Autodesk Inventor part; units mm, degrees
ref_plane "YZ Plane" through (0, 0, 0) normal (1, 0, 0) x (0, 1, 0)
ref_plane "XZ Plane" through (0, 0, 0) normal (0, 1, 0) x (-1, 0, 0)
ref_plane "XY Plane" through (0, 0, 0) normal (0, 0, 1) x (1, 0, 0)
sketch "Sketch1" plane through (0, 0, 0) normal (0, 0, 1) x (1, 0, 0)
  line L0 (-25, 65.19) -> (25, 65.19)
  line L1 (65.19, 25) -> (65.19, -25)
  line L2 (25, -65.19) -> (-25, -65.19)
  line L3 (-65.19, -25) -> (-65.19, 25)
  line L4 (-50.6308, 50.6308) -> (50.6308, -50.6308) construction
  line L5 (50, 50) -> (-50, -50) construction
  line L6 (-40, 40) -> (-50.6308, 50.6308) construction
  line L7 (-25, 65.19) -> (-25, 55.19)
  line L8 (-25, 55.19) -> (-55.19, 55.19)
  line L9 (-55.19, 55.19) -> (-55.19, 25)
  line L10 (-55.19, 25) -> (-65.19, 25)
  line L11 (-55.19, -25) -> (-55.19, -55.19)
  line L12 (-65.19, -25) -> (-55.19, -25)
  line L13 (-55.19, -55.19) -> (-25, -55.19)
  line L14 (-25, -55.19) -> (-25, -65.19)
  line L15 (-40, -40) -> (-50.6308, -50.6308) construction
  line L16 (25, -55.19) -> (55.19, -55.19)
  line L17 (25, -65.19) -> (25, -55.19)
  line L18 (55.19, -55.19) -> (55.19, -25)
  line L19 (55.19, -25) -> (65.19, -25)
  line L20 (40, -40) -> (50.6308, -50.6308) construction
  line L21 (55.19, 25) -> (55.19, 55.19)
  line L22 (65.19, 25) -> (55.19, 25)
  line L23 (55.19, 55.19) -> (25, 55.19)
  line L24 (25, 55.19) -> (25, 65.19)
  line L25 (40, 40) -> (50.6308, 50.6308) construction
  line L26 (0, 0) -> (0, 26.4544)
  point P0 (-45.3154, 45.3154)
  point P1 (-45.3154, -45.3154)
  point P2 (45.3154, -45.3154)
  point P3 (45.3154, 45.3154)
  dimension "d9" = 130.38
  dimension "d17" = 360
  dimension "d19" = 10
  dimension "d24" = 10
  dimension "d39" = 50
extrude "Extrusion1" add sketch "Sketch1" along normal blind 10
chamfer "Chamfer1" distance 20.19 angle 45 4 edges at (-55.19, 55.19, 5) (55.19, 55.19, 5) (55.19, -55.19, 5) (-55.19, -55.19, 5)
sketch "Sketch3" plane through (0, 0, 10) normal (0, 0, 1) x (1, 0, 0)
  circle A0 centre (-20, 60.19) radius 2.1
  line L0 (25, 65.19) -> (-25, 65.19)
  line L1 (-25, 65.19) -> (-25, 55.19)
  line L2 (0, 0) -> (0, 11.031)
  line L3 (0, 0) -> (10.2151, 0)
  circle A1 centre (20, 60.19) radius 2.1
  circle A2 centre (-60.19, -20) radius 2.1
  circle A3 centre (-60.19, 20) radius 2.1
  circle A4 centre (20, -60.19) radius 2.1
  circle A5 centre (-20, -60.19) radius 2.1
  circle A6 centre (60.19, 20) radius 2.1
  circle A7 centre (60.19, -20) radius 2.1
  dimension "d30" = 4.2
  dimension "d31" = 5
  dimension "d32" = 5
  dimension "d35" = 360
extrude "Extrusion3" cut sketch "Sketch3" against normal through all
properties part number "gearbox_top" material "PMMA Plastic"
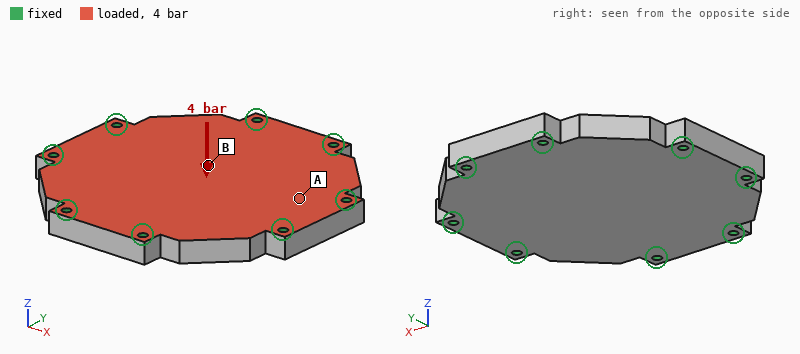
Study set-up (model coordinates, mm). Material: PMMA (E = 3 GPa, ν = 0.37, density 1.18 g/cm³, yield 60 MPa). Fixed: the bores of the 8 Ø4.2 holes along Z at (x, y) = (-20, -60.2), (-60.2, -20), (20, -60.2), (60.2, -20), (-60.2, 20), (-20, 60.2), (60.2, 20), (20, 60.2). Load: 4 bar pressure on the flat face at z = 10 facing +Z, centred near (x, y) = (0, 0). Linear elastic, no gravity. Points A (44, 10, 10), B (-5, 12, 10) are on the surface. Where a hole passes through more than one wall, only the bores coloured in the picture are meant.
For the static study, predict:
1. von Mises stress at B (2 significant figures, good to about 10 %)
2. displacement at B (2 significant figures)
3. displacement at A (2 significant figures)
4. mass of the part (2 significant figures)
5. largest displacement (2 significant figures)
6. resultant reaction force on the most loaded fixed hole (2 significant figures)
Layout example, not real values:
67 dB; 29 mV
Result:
10 MPa; 0.61 mm; 0.24 mm; 160 g; 0.65 mm; 660 N
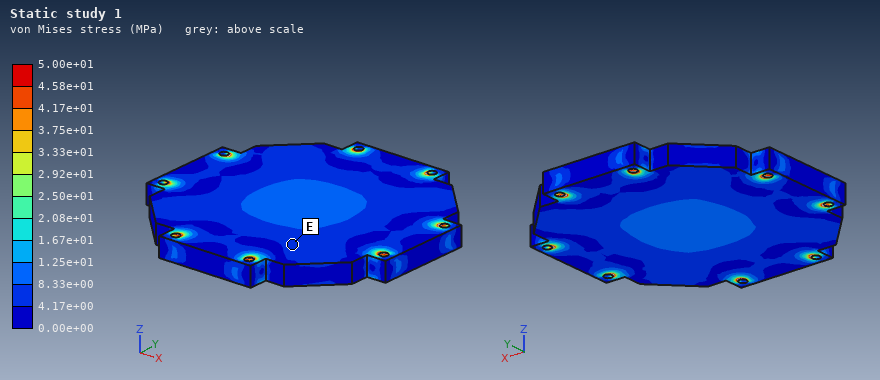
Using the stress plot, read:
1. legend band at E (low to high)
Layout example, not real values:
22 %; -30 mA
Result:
4.17e+00 to 8.33e+00 MPa
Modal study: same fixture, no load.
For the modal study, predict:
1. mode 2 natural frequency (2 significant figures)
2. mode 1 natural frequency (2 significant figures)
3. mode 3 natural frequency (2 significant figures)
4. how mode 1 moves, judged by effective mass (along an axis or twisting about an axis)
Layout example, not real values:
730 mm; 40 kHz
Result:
2900 Hz; 1400 Hz; 2900 Hz; along Z
